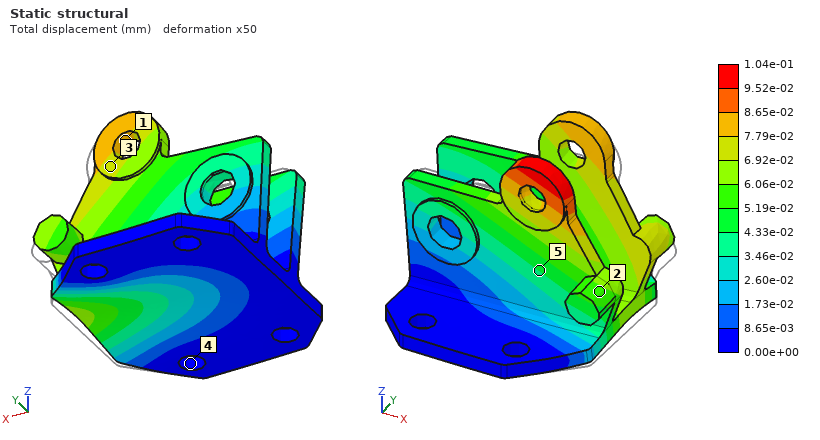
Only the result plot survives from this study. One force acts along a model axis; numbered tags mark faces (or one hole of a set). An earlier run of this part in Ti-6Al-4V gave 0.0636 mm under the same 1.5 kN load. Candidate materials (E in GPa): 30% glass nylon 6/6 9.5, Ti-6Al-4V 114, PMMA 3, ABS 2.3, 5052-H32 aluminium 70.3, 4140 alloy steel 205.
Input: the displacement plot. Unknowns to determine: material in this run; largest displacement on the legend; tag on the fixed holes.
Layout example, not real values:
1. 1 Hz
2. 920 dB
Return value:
1. 5052-H32 aluminium
2. 1.04e-01 mm
3. 4
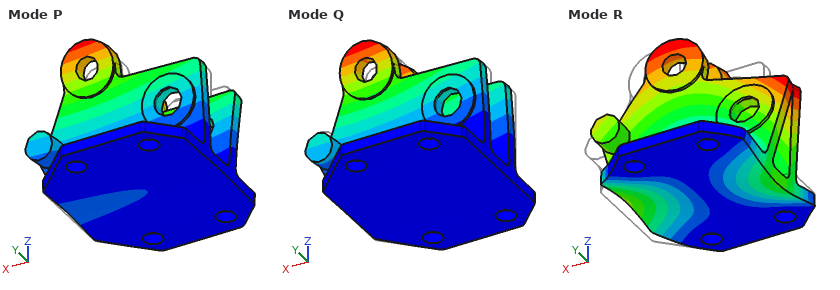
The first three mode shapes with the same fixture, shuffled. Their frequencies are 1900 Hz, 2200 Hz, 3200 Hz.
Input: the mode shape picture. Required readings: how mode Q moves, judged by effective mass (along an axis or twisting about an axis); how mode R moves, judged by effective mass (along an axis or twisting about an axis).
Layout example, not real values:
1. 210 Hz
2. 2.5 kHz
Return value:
1. along Y
2. along X
